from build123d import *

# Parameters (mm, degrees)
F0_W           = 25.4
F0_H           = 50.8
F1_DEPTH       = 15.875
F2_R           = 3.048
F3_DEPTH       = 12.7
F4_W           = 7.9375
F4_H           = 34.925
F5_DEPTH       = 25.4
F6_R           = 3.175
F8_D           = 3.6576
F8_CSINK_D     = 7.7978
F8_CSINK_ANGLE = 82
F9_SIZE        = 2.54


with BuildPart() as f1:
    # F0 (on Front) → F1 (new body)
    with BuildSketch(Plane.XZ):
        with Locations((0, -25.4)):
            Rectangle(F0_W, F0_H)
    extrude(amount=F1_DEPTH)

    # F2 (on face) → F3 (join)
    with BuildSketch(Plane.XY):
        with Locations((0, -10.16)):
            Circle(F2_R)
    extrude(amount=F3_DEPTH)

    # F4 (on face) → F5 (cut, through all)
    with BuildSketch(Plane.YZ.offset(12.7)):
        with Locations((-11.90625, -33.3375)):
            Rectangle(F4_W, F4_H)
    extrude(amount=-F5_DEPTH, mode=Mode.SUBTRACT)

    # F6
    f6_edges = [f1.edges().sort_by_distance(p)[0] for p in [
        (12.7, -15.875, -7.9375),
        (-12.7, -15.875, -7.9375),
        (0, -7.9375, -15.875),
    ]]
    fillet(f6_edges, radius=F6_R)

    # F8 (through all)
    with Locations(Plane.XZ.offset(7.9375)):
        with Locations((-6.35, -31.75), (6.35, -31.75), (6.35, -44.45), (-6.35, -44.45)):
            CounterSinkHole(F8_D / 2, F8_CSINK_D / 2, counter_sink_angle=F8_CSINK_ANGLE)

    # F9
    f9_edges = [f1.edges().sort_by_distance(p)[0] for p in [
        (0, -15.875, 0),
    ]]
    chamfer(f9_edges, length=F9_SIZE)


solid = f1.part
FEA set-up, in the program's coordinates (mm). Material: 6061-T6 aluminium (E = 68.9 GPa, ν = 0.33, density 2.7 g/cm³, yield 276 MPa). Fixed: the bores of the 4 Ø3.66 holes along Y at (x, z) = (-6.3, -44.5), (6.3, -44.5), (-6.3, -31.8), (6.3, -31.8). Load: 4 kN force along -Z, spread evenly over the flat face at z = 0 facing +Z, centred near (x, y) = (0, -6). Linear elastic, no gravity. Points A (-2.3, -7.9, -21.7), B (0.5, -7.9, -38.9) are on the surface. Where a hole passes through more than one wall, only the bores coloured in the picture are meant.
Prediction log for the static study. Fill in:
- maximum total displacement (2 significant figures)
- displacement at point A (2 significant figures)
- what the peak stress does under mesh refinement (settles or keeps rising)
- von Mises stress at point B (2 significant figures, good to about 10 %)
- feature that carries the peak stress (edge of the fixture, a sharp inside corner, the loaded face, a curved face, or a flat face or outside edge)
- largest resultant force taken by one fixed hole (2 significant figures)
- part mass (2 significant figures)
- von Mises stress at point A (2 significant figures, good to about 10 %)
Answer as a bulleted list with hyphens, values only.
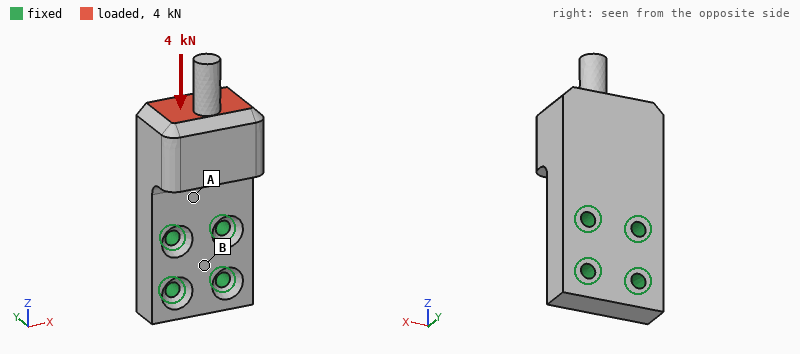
- 99 µm
- 16 µm
- keeps rising
- 12 MPa
- edge of the fixture
- 1.6 kN
- 35 g
- 53 MPa
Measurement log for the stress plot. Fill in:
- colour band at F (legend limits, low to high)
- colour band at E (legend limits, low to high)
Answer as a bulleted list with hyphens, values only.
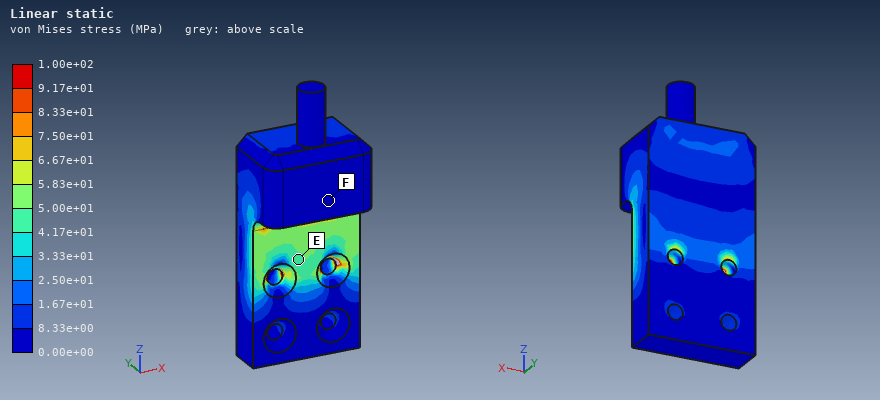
- 0.00e+00 to 8.33e+00 MPa
- 4.17e+01 to 5.00e+01 MPa
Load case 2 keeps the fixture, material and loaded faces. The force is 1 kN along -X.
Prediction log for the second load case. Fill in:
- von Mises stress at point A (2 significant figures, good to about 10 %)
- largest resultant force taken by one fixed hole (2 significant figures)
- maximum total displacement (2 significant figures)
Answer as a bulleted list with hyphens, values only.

- 17 MPa
- 1.7 kN
- 33 µm
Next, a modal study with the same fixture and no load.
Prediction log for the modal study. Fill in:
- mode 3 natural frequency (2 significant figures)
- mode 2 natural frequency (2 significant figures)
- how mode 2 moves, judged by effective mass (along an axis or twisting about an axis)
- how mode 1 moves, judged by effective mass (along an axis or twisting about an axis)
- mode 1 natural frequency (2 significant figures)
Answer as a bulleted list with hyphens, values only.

- 12 kHz
- 8800 Hz
- along X
- along Y
- 3700 Hz
